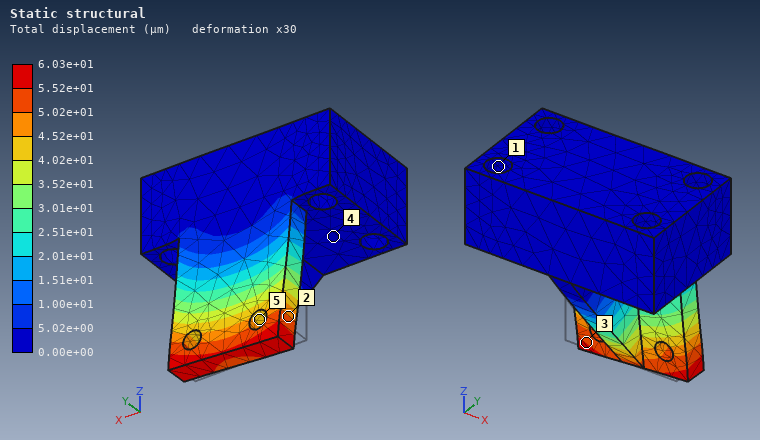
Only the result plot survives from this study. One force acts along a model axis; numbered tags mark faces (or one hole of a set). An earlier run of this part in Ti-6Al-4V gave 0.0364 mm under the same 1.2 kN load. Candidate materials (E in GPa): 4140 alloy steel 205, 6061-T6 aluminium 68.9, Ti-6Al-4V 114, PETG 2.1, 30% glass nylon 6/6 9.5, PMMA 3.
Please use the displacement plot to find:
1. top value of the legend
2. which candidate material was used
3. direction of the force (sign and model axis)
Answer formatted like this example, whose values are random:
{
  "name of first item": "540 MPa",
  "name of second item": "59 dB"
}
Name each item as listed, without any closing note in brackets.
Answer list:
{
  "top value of the legend": "6.03e+01 µm",
  "which candidate material was used": "6061-T6 aluminium",
  "direction of the force": "+X"
}
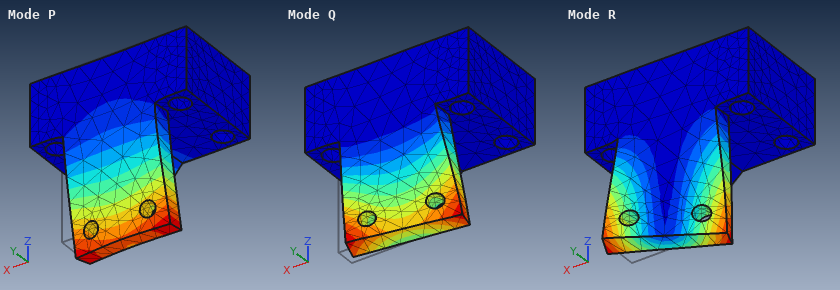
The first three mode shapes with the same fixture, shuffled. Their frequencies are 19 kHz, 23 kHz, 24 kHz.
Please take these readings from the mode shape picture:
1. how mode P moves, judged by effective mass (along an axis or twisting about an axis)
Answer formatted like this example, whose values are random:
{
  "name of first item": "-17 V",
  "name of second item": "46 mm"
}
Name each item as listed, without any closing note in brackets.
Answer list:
{
  "how mode P moves, judged by effective mass": "along Y"
}
